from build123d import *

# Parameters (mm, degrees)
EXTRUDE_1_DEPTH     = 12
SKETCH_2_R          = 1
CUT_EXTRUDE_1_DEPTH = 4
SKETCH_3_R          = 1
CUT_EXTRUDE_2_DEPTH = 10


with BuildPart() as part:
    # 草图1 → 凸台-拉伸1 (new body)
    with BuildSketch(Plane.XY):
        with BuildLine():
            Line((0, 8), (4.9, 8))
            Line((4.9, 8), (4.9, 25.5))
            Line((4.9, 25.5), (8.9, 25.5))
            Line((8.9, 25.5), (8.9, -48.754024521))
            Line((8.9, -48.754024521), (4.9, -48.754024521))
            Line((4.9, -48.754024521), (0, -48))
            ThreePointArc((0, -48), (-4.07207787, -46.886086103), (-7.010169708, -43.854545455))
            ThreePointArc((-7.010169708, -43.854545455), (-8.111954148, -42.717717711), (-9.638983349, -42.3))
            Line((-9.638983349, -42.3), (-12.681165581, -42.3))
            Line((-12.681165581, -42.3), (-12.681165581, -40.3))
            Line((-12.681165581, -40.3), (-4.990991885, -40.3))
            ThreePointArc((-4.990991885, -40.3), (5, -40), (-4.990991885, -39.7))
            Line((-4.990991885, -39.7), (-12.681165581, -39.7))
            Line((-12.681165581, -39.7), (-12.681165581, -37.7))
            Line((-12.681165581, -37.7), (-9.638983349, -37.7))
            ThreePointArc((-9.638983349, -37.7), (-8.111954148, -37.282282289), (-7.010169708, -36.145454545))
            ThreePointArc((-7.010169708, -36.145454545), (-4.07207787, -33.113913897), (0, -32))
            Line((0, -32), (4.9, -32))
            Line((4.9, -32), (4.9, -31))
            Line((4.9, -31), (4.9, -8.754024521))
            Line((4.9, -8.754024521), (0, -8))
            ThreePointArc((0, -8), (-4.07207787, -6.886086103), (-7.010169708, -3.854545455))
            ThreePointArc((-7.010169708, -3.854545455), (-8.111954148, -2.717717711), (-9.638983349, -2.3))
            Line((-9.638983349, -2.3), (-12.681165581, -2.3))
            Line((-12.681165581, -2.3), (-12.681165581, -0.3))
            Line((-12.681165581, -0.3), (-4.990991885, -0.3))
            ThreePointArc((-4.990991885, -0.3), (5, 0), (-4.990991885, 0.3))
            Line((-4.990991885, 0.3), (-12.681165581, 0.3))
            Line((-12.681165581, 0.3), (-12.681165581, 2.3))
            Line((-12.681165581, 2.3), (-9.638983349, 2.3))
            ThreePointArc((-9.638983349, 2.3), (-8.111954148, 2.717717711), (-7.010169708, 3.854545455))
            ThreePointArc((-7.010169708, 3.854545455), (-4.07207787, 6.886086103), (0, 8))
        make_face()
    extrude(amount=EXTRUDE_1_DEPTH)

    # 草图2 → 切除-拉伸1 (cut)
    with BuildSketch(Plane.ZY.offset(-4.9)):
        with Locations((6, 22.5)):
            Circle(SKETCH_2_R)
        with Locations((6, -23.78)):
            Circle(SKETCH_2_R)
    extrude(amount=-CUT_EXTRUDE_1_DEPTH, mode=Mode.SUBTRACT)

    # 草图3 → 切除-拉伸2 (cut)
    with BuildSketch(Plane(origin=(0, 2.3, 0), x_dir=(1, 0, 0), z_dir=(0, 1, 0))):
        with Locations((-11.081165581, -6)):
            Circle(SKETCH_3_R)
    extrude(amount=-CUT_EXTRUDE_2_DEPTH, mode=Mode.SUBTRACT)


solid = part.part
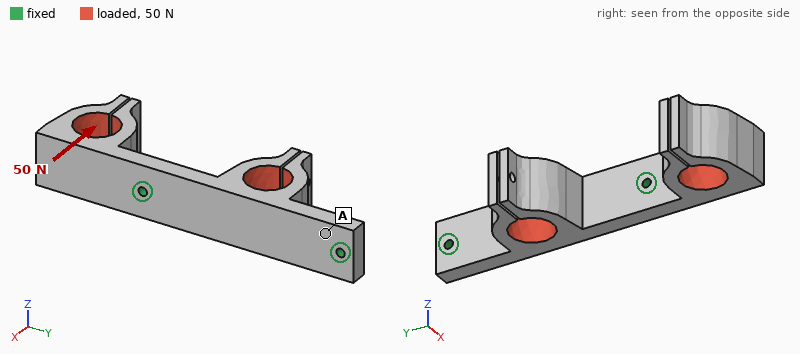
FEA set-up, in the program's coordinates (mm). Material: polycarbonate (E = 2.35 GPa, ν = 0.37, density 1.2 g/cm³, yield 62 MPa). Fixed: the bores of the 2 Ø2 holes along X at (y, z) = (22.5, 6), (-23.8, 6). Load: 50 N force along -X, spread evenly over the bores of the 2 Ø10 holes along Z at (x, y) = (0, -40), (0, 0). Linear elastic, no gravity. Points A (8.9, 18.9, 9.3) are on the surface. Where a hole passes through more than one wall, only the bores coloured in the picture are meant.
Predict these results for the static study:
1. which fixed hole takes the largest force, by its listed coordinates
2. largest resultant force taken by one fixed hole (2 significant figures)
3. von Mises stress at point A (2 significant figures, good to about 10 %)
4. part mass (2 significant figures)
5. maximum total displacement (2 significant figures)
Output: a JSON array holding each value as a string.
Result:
["(-23.8, 6)", "39 N", "1.8 MPa", "7.7 g", "0.50 mm"]
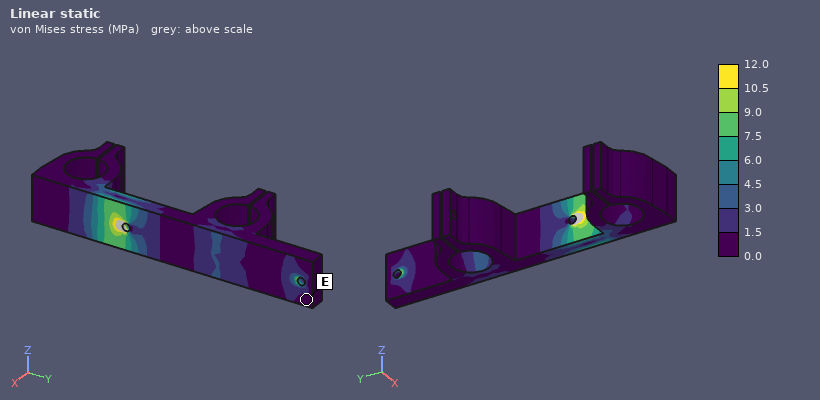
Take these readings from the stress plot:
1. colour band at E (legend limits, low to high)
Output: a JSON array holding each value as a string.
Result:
["0.0 to 1.5 MPa"]
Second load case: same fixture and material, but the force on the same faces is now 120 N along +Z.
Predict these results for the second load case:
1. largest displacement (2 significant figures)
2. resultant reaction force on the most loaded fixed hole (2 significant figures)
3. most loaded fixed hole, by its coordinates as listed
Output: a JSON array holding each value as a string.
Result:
["0.76 mm", "100 N", "(-23.8, 6)"]
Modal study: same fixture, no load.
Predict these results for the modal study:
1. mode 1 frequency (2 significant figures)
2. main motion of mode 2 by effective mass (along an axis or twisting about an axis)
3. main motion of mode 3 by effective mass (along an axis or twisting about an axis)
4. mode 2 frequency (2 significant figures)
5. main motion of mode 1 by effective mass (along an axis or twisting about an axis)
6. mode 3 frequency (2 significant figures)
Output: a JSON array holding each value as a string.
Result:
["700 Hz", "along Z", "along Z", "1100 Hz", "along X", "1400 Hz"]
